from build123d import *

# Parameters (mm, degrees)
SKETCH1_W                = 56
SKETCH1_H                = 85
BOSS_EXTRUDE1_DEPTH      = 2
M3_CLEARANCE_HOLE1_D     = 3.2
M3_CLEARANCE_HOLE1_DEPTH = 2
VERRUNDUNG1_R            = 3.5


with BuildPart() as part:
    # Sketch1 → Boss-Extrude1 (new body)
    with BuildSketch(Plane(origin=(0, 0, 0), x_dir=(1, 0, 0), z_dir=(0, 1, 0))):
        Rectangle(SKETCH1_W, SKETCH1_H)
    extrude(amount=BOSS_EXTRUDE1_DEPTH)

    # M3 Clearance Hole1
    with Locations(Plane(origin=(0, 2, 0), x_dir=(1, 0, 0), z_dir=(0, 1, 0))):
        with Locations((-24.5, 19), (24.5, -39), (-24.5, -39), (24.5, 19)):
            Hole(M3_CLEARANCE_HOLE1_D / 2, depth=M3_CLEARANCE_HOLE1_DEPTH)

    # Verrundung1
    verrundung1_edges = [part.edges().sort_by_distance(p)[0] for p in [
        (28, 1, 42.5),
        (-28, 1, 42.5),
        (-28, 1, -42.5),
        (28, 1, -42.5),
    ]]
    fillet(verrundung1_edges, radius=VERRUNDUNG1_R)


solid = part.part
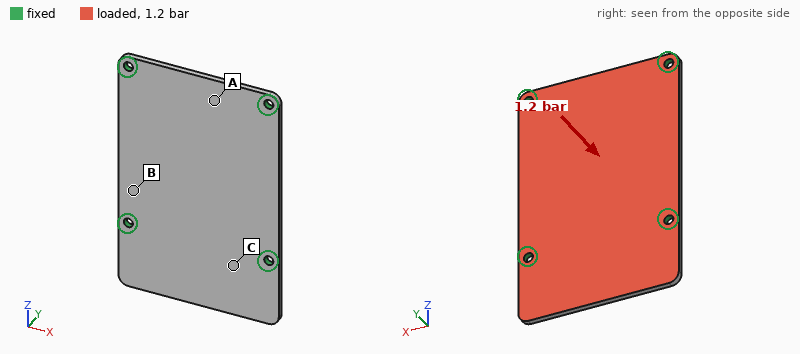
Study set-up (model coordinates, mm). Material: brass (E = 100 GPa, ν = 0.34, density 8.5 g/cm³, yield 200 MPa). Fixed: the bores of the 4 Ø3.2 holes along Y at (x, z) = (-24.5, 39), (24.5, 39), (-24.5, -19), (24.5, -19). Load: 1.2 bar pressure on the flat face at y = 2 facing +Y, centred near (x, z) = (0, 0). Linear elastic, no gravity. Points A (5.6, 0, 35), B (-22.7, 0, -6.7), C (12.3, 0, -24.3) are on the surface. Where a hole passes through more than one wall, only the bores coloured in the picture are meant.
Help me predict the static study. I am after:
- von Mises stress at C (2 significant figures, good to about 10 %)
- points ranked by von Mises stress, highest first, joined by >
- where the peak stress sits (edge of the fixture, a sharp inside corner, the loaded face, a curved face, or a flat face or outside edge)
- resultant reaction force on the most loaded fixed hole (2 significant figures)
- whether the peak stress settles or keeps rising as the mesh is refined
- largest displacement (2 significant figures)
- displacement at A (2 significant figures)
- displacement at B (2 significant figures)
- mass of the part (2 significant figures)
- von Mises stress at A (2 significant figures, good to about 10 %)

30 MPa
C > A > B
edge of the fixture
180 N
keeps rising
0.11 mm
0.044 mm
0.030 mm
80 g
20 MPa
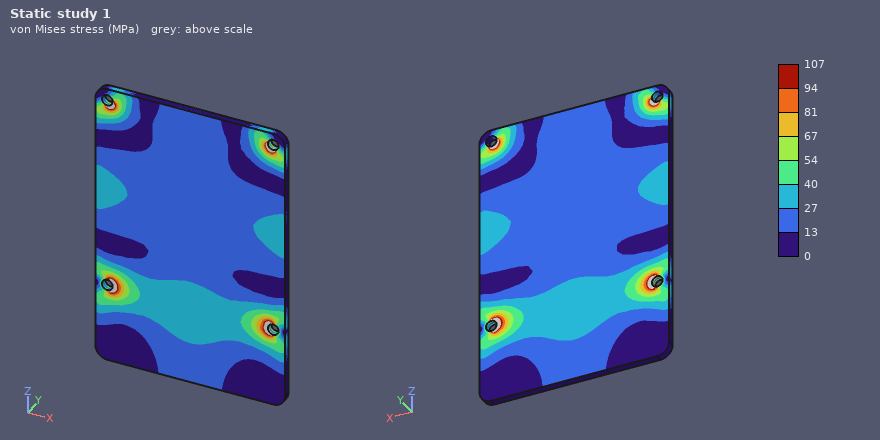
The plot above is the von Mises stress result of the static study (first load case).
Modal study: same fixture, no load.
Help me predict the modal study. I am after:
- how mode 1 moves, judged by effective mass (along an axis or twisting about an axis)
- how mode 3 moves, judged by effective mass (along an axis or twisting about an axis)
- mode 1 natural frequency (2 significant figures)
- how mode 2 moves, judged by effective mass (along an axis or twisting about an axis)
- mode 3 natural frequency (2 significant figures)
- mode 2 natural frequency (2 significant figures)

twisting about X
twisting about Z
1400 Hz
along Y
2500 Hz
1700 Hz
